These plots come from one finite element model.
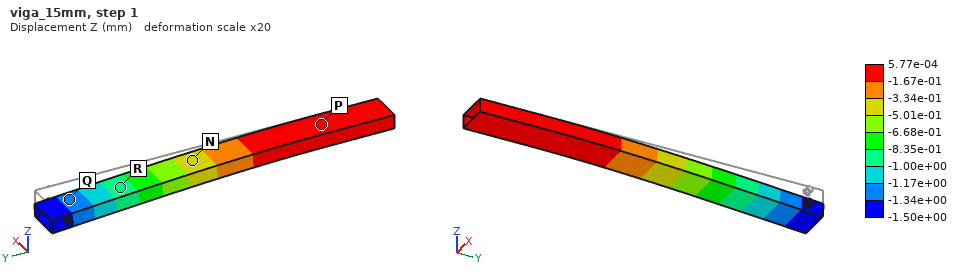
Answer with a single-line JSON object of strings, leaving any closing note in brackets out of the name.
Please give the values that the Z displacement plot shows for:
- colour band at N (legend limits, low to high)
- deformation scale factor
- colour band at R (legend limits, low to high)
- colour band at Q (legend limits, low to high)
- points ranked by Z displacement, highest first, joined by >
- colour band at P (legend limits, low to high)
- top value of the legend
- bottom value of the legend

{"colour band at N": "-5.01e-01 to -3.34e-01 mm", "deformation scale factor": "20", "colour band at R": "-1.00e+00 to -8.35e-01 mm", "colour band at Q": "-1.34e+00 to -1.17e+00 mm", "points ranked by Z displacement, highest first, joined by >": "P > N > R > Q", "colour band at P": "-1.67e-01 to 5.77e-04 mm", "top value of the legend": "5.77e-04 mm", "bottom value of the legend": "-1.50e+00 mm"}
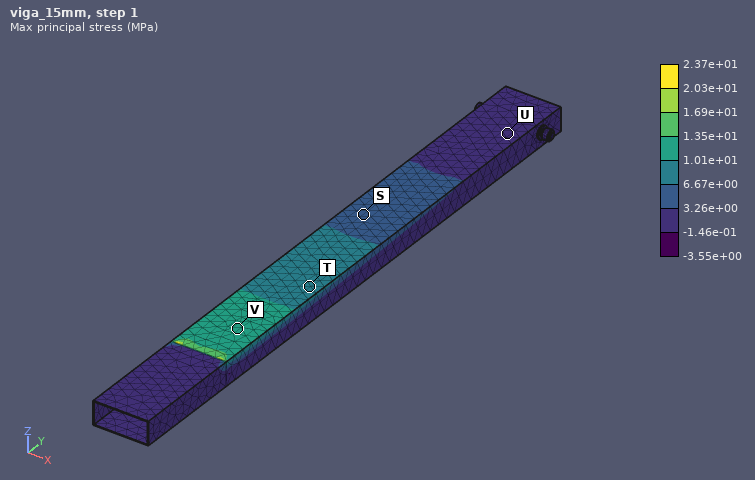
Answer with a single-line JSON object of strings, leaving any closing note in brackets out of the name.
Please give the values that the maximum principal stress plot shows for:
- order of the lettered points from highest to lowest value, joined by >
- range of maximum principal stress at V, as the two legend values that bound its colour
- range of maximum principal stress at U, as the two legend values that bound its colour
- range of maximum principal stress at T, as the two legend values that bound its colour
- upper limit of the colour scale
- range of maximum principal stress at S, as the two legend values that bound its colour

{"order of the lettered points from highest to lowest value, joined by >": "V > T > S > U", "range of maximum principal stress at V, as the two legend values that bound its colour": "1.01e+01 to 1.35e+01 MPa", "range of maximum principal stress at U, as the two legend values that bound its colour": "-1.46e-01 to 3.26e+00 MPa", "range of maximum principal stress at T, as the two legend values that bound its colour": "6.67e+00 to 1.01e+01 MPa", "upper limit of the colour scale": "2.37e+01 MPa", "range of maximum principal stress at S, as the two legend values that bound its colour": "3.26e+00 to 6.67e+00 MPa"}
